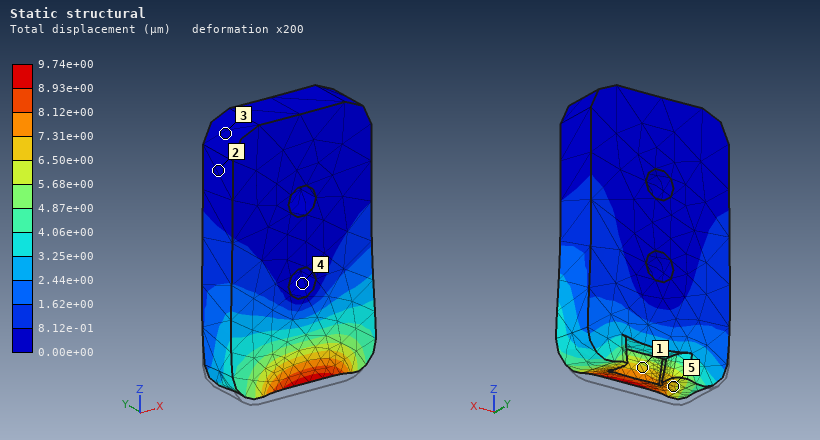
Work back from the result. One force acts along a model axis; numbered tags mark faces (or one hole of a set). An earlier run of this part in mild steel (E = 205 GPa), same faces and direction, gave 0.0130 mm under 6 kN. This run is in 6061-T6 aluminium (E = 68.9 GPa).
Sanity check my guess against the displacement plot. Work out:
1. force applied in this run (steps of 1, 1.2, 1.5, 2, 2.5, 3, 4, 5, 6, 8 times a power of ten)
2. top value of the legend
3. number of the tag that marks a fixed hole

1.5 kN
9.74e+00 µm
4
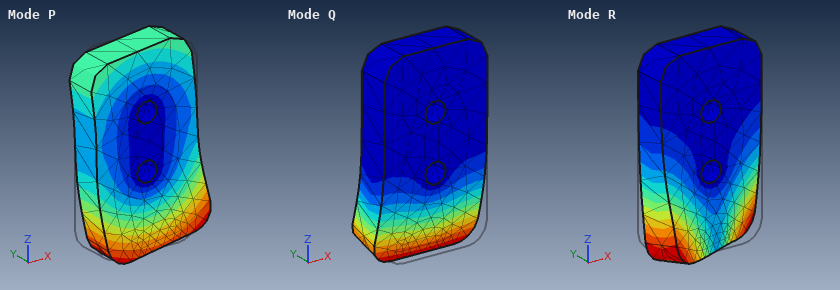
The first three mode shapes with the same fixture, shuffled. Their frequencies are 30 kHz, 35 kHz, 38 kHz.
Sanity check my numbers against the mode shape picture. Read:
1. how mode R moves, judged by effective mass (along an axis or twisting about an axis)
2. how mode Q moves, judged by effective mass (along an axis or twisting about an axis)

twisting about Z
along Y
